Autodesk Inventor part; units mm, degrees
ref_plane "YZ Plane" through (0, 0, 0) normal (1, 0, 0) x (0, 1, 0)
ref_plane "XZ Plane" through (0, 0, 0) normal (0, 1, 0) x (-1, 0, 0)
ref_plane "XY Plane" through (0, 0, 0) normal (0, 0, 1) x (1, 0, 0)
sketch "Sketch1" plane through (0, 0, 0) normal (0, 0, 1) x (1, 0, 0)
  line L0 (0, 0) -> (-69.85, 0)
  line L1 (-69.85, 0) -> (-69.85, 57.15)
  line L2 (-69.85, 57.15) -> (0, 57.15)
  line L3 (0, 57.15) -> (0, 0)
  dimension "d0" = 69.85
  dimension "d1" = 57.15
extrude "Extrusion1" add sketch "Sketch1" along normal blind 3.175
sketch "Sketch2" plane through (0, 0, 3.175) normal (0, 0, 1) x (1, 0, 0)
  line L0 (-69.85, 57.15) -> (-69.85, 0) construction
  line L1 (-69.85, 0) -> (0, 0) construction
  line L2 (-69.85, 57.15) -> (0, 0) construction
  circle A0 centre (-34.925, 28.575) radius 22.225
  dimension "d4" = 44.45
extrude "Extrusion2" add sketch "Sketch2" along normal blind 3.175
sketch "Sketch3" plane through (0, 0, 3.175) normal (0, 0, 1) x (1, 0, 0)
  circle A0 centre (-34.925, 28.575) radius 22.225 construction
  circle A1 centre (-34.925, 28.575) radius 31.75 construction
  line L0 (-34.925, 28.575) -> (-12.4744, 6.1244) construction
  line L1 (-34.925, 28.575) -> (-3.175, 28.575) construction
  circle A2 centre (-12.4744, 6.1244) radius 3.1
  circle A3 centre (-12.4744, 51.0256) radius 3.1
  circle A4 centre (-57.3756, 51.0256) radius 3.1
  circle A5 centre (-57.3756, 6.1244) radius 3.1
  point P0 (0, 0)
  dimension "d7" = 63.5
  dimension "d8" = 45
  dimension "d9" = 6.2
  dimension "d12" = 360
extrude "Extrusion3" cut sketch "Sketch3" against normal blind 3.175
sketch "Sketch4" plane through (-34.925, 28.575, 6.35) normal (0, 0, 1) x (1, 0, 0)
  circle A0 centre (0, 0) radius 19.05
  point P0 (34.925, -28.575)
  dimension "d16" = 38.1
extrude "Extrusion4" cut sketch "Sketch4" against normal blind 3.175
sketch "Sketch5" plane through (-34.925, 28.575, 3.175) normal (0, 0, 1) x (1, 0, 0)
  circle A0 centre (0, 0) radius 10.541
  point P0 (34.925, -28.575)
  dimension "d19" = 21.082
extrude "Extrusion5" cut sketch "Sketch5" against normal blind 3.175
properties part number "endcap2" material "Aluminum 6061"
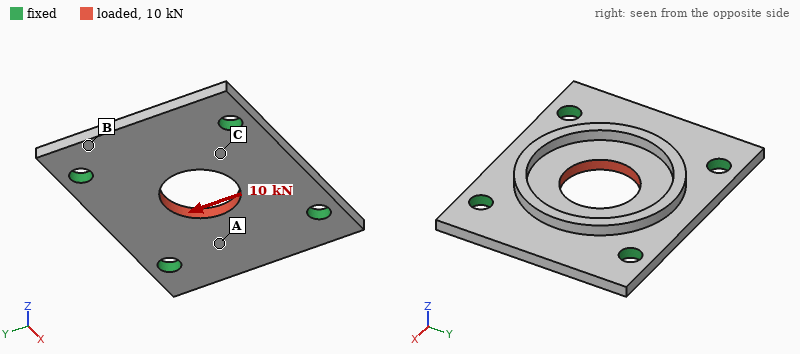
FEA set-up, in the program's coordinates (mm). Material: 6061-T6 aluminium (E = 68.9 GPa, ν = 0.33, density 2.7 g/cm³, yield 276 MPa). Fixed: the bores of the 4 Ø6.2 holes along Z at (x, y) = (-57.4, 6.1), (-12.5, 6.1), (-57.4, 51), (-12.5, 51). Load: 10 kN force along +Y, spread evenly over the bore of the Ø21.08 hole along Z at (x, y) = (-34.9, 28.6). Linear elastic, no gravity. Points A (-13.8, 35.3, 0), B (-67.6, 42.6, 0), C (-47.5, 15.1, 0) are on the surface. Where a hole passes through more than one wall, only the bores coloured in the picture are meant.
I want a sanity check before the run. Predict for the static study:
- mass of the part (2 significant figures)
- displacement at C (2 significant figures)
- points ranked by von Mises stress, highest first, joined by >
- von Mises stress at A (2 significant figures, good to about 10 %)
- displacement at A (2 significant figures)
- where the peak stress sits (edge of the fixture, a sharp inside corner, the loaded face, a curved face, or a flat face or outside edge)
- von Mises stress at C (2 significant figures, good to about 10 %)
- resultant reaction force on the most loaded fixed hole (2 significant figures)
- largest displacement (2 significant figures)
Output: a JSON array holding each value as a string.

["34 g", "13 µm", "C > A > B", "30 MPa", "7.2 µm", "edge of the fixture", "53 MPa", "2.7 kN", "27 µm"]
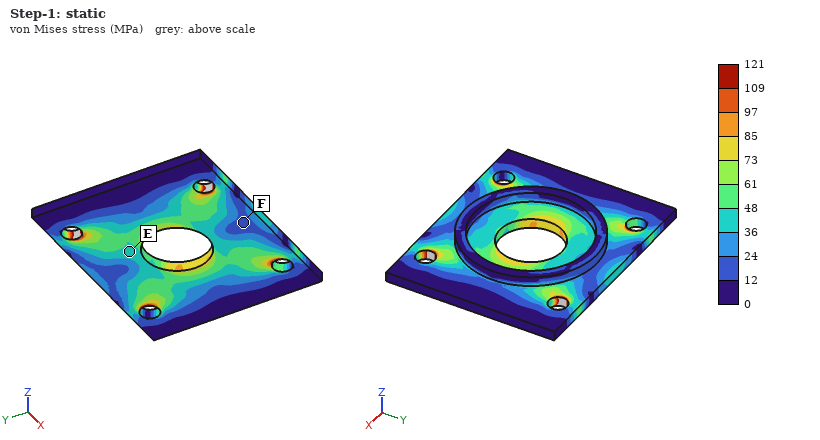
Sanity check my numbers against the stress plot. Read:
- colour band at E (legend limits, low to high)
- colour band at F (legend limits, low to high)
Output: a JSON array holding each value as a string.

["36 to 48 MPa", "12 to 24 MPa"]
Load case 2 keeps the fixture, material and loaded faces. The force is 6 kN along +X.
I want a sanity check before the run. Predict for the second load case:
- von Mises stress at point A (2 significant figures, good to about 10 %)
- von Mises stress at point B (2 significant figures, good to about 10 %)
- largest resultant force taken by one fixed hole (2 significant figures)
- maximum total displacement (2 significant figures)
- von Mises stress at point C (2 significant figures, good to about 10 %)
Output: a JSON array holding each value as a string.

["20 MPa", "10 MPa", "1.6 kN", "14 µm", "28 MPa"]
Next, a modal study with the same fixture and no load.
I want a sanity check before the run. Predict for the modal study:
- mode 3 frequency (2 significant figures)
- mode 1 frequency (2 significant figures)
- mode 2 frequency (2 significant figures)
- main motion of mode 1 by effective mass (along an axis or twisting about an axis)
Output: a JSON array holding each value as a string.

["9400 Hz", "8300 Hz", "9400 Hz", "along Z"]
